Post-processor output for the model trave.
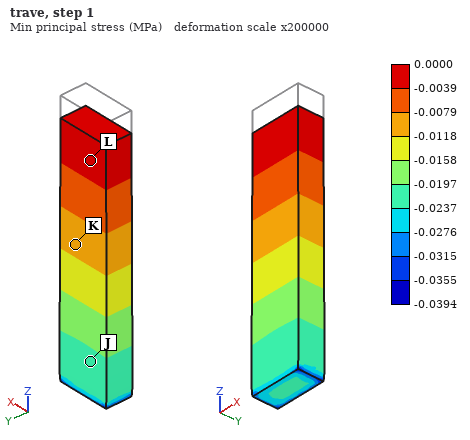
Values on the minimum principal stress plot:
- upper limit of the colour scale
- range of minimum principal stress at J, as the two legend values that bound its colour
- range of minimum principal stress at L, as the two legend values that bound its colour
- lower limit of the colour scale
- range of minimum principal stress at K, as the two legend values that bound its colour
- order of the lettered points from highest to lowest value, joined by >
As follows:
0.0000 MPa
-0.0237 to -0.0197 MPa
-0.0039 to 0.0000 MPa
-0.0394 MPa
-0.0118 to -0.0079 MPa
L > K > J
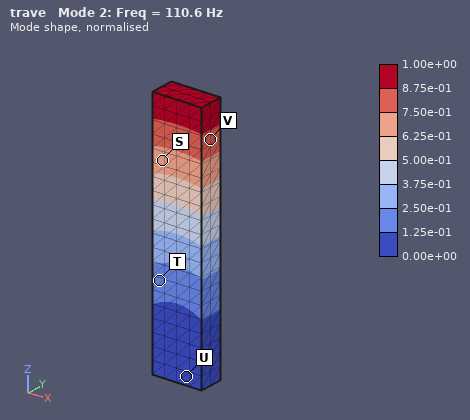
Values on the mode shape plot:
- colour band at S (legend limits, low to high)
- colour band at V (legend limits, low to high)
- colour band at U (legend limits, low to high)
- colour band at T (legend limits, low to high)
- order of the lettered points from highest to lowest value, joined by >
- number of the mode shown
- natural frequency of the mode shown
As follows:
6.25e-01 to 7.50e-01
7.50e-01 to 8.75e-01
0.00e+00 to 1.25e-01
1.25e-01 to 2.50e-01
V > S > T > U
2
110.6 Hz
